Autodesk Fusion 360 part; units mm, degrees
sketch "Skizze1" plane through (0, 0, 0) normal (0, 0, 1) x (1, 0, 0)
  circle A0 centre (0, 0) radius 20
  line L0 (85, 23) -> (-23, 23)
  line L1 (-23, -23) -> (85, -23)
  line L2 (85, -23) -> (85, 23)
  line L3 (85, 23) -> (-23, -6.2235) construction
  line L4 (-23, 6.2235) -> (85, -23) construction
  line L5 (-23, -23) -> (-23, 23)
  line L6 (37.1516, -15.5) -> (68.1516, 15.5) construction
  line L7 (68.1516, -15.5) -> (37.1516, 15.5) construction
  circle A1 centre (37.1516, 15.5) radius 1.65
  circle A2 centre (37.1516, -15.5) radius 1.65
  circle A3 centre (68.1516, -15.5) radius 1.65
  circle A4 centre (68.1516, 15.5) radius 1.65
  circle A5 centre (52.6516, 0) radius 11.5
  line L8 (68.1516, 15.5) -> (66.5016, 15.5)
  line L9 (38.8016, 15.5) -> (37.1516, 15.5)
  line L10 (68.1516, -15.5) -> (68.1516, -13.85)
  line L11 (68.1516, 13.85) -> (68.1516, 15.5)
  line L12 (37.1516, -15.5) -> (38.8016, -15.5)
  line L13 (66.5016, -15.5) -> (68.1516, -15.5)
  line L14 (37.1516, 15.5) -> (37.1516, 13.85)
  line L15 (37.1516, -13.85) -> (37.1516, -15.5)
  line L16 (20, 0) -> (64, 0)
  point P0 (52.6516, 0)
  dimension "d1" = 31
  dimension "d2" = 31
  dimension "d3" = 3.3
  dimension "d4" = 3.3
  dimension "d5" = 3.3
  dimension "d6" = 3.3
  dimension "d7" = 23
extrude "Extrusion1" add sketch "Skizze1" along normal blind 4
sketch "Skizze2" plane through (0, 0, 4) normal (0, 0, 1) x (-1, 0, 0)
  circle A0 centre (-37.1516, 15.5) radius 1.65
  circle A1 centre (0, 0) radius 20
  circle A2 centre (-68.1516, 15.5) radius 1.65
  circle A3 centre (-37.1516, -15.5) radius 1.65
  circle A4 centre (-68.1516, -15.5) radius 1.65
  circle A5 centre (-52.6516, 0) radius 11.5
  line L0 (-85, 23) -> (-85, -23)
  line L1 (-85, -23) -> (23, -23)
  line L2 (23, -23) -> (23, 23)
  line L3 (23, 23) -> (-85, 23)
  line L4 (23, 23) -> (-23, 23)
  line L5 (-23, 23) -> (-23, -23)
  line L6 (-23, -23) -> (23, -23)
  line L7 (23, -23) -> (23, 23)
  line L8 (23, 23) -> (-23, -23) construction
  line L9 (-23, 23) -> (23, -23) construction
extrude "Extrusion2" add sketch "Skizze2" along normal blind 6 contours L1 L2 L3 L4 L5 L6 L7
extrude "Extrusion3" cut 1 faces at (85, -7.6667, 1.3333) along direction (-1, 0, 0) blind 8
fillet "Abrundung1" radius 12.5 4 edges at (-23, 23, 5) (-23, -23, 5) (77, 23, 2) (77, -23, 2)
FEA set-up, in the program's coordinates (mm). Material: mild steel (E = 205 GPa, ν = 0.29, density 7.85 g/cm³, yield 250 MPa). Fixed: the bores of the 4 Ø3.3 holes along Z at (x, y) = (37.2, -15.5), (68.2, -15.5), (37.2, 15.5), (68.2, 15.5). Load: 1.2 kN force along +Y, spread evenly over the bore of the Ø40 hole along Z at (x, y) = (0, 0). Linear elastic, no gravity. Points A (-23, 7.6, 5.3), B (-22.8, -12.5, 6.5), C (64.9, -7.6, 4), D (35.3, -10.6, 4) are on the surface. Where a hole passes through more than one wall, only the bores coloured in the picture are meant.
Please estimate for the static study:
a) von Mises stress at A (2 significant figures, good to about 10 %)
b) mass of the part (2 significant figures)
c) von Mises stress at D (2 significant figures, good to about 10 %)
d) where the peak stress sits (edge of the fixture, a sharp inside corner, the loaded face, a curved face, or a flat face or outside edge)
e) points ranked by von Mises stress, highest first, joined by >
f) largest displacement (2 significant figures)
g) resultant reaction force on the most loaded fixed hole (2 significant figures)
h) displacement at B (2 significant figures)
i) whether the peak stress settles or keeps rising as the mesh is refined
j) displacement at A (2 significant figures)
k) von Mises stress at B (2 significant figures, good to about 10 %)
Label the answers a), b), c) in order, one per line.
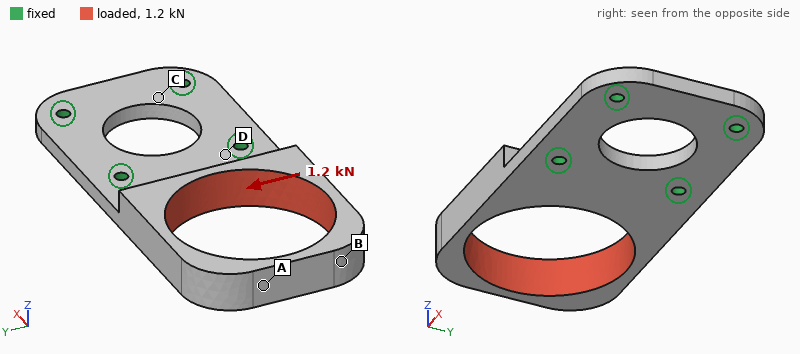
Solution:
a) 42 MPa
b) 120 g
c) 22 MPa
d) edge of the fixture
e) A > B > D > C
f) 61 µm
g) 1.3 kN
h) 61 µm
i) keeps rising
j) 60 µm
k) 29 MPa
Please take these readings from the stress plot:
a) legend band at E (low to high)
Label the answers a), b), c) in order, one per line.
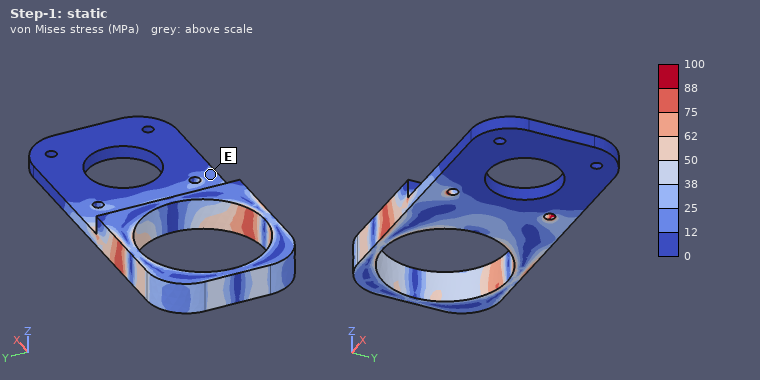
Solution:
a) 12 to 25 MPa
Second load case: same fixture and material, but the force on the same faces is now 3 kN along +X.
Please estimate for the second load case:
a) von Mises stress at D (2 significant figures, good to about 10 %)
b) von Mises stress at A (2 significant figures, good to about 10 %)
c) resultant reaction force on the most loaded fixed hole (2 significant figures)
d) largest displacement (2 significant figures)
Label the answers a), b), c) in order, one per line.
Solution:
a) 64 MPa
b) 30 MPa
c) 1.4 kN
d) 0.18 mm
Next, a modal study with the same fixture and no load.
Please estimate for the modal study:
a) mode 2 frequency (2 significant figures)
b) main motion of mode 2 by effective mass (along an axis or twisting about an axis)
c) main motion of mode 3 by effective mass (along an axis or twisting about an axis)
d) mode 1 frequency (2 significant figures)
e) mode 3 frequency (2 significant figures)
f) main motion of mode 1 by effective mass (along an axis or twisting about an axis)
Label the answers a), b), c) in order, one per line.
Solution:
a) 2500 Hz
b) twisting about X
c) along Y
d) 970 Hz
e) 3200 Hz
f) along Z
